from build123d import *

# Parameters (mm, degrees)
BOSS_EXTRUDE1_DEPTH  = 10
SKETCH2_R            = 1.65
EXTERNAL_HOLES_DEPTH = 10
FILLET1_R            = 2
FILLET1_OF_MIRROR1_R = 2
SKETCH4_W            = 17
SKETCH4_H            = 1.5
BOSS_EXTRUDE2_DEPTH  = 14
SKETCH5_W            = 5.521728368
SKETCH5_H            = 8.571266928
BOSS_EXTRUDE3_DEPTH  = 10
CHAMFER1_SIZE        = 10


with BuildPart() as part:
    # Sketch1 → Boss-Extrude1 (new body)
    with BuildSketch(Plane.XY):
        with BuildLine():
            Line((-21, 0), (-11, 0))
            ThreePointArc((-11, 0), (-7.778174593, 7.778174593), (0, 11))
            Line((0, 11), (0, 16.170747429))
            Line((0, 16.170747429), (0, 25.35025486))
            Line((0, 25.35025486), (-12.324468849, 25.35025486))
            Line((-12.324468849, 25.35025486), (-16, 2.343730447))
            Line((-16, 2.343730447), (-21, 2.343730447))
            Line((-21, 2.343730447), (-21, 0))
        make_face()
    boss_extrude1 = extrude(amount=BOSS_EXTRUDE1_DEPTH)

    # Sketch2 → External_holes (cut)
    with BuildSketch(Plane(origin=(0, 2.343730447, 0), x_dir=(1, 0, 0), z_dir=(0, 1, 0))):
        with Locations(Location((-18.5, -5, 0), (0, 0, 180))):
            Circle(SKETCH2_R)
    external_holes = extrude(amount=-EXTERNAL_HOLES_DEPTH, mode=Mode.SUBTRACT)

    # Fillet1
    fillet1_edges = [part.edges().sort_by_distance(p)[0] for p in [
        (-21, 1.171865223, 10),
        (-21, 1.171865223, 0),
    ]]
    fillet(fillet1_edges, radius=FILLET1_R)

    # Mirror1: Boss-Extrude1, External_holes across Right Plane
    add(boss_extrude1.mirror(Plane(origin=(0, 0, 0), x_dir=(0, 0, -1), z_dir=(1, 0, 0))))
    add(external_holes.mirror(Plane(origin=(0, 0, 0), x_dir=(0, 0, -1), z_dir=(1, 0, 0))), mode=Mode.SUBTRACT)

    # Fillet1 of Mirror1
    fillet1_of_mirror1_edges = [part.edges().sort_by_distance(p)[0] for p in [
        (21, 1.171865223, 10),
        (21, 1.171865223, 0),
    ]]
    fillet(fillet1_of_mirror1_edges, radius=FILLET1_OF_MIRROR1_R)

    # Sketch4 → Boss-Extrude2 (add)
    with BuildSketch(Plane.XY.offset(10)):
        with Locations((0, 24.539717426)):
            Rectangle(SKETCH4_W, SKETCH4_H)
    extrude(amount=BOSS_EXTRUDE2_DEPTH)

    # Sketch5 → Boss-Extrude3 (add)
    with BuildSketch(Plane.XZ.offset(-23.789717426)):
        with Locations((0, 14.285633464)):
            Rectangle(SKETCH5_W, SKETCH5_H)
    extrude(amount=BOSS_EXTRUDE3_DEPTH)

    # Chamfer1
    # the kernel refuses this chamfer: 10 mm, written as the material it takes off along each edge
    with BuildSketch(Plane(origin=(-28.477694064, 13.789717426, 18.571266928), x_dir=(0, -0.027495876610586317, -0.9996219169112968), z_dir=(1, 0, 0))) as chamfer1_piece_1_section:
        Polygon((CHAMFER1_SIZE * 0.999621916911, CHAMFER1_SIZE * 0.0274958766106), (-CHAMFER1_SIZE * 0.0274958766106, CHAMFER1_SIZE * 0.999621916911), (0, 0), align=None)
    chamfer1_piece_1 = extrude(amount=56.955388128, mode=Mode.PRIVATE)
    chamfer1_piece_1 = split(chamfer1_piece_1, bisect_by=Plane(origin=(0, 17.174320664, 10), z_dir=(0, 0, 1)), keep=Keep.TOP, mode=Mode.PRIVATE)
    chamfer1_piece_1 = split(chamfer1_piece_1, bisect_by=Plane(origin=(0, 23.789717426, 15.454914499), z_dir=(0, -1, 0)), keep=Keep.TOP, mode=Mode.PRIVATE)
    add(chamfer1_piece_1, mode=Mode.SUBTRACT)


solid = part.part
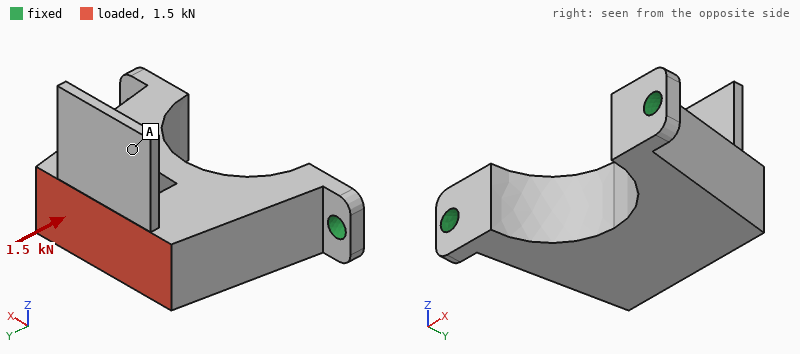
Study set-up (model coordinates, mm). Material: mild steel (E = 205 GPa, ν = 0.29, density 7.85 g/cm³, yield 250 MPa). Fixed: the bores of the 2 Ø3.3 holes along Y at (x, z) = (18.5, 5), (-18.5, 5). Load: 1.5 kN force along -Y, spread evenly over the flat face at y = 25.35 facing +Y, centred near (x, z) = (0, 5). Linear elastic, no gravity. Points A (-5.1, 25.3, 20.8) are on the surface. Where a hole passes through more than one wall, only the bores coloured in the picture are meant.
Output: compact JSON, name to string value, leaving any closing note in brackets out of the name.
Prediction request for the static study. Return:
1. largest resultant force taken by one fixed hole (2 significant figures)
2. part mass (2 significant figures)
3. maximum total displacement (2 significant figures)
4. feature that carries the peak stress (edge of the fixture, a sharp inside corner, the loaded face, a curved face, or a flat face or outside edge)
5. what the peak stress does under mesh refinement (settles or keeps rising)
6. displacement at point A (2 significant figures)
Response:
{"largest resultant force taken by one fixed hole": "870 N", "part mass": "48 g", "maximum total displacement": "3.8 µm", "feature that carries the peak stress": "edge of the fixture", "what the peak stress does under mesh refinement": "keeps rising", "displacement at point A": "3.7 µm"}
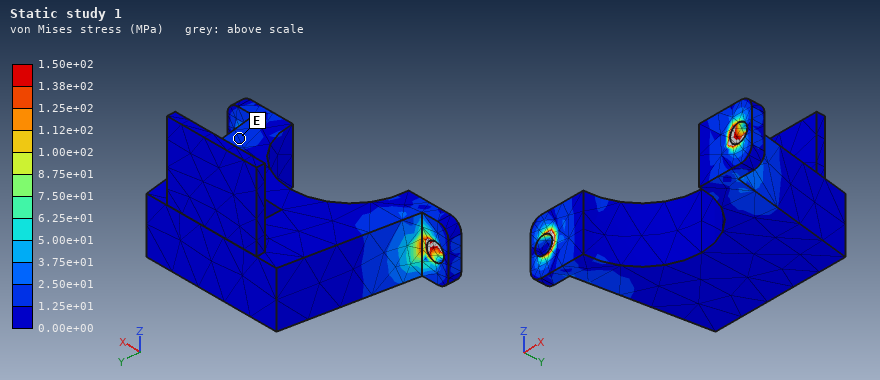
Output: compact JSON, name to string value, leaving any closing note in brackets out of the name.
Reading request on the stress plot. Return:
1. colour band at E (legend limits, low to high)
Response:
{"colour band at E": "1.25e+01 to 2.50e+01 MPa"}
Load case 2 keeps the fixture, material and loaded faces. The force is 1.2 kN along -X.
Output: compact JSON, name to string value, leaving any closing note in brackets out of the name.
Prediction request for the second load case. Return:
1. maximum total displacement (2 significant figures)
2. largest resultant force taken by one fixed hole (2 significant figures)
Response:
{"maximum total displacement": "7.8 µm", "largest resultant force taken by one fixed hole": "1.1 kN"}
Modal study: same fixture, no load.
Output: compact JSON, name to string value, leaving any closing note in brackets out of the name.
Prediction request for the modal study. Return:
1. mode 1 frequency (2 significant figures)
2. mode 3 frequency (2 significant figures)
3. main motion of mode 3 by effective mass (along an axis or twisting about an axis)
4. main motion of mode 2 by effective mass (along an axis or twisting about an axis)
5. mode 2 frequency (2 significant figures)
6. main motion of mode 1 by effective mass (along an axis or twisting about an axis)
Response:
{"mode 1 frequency": "2400 Hz", "mode 3 frequency": "14 kHz", "main motion of mode 3 by effective mass": "along X", "main motion of mode 2 by effective mass": "along X", "mode 2 frequency": "12 kHz", "main motion of mode 1 by effective mass": "along Z"}
